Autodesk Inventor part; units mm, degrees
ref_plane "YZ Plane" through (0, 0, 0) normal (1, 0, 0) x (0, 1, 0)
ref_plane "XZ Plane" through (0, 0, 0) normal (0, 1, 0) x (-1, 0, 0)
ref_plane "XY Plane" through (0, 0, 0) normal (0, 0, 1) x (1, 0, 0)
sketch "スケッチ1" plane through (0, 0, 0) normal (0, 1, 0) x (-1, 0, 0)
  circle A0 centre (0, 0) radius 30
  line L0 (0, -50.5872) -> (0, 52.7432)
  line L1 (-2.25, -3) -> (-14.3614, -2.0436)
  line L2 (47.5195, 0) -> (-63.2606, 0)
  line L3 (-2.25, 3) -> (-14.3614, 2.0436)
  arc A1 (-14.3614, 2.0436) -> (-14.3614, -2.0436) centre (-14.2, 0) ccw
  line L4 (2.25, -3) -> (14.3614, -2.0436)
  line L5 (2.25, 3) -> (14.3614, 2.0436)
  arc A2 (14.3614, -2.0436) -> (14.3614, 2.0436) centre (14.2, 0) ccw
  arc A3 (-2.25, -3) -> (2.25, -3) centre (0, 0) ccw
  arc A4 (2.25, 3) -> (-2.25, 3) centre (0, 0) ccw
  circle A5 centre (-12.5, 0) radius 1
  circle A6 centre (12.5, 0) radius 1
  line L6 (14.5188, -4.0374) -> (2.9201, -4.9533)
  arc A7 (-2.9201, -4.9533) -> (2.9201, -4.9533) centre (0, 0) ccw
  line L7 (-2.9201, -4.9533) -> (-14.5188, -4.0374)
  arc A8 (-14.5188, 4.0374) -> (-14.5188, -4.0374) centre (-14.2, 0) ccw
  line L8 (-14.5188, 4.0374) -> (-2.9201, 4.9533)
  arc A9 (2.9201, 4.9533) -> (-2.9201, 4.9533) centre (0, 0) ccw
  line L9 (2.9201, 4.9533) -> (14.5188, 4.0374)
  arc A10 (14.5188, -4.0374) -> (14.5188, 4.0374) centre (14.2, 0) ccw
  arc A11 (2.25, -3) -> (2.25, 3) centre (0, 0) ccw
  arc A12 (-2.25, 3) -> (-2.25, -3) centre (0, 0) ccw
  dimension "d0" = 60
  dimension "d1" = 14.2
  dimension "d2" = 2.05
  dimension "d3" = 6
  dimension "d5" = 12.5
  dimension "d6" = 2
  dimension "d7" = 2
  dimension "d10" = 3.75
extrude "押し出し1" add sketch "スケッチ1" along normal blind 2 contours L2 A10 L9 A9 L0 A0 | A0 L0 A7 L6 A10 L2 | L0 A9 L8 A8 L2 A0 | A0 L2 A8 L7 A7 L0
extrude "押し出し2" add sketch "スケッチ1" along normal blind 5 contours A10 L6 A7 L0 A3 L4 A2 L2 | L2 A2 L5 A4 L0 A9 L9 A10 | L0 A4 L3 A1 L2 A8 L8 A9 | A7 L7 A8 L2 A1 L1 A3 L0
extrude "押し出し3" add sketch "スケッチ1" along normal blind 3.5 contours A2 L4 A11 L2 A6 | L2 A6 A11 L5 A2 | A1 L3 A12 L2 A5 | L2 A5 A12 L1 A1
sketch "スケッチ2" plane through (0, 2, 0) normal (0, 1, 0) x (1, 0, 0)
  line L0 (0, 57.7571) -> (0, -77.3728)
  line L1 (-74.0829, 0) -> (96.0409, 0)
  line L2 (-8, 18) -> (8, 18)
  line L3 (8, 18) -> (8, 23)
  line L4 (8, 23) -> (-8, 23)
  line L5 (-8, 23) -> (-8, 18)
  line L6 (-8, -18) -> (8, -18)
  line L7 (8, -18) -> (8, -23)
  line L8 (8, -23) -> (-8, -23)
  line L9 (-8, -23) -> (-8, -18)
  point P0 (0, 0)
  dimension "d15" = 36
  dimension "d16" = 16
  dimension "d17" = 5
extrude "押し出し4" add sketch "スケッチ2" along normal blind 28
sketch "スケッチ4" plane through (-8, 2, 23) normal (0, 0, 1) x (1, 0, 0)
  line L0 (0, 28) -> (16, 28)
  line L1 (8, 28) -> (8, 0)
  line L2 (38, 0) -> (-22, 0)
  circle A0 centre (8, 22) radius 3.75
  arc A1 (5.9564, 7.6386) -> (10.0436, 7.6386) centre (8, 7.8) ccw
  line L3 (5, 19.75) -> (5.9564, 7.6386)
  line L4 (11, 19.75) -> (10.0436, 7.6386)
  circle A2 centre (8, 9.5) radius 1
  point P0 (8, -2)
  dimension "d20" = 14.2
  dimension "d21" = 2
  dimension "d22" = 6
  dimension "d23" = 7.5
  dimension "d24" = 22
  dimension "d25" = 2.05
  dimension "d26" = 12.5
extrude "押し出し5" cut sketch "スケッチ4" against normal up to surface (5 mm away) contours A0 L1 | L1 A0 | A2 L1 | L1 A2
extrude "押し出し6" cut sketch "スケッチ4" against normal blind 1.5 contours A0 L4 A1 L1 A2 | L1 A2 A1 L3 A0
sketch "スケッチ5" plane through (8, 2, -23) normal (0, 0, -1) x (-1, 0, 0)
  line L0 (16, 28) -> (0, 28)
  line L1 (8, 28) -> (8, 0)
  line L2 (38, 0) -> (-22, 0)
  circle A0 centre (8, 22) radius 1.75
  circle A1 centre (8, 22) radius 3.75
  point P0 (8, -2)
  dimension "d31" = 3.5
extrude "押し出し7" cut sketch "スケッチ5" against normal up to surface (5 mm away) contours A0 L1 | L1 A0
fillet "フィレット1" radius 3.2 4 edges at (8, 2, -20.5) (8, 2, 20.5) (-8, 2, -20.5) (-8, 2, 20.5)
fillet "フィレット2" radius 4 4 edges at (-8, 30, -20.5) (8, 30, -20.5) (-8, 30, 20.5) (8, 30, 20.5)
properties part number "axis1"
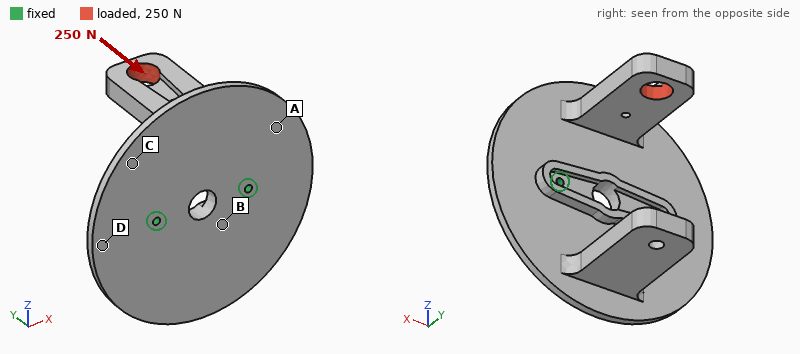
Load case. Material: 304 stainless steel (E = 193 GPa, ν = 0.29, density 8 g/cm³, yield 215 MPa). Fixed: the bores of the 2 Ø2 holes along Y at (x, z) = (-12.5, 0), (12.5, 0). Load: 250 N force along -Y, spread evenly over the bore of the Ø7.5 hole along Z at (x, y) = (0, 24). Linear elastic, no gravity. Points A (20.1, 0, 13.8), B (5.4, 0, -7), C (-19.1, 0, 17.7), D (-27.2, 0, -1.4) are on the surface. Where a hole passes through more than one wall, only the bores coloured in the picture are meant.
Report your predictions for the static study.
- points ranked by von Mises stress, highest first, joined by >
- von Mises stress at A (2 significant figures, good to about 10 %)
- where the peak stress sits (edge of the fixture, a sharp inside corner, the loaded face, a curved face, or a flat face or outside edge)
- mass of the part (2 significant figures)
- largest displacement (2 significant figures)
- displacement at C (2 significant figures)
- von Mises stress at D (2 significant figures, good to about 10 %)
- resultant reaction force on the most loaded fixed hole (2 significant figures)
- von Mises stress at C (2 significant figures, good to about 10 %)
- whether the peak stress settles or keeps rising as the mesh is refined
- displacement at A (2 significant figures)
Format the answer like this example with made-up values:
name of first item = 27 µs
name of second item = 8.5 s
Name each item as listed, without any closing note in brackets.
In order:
points ranked by von Mises stress, highest first, joined by > = A > C > D > B
von Mises stress at A = 53 MPa
where the peak stress sits = edge of the fixture
mass of the part = 82 g
largest displacement = 0.21 mm
displacement at C = 0.058 mm
von Mises stress at D = 21 MPa
resultant reaction force on the most loaded fixed hole = 130 N
von Mises stress at C = 39 MPa
whether the peak stress settles or keeps rising as the mesh is refined = keeps rising
displacement at A = 0.037 mm
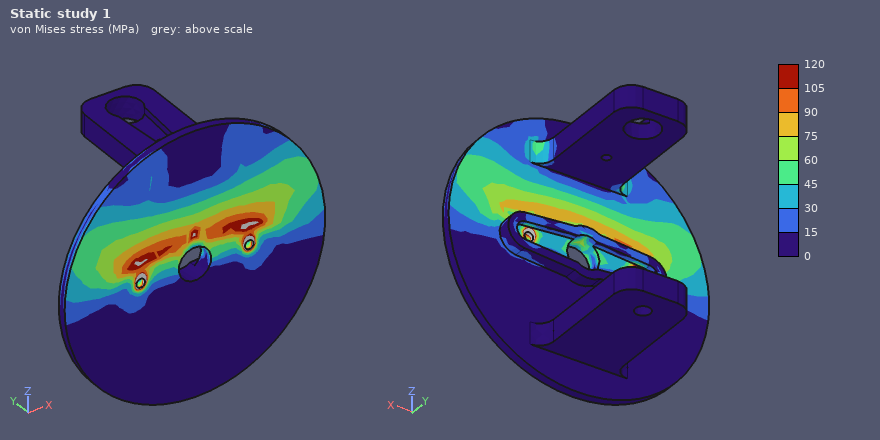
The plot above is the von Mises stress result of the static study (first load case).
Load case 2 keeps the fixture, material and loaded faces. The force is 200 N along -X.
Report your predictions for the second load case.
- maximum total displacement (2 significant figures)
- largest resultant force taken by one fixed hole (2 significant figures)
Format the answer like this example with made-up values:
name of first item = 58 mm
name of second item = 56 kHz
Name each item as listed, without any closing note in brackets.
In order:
maximum total displacement = 0.11 mm
largest resultant force taken by one fixed hole = 250 N
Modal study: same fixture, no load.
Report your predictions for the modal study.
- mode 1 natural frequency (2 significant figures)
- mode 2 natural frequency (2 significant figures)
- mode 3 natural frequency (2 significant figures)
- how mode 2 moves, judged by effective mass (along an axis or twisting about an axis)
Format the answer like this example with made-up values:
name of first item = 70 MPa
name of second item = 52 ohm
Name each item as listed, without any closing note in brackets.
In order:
mode 1 natural frequency = 1100 Hz
mode 2 natural frequency = 1200 Hz
mode 3 natural frequency = 2200 Hz
how mode 2 moves, judged by effective mass = along Y
